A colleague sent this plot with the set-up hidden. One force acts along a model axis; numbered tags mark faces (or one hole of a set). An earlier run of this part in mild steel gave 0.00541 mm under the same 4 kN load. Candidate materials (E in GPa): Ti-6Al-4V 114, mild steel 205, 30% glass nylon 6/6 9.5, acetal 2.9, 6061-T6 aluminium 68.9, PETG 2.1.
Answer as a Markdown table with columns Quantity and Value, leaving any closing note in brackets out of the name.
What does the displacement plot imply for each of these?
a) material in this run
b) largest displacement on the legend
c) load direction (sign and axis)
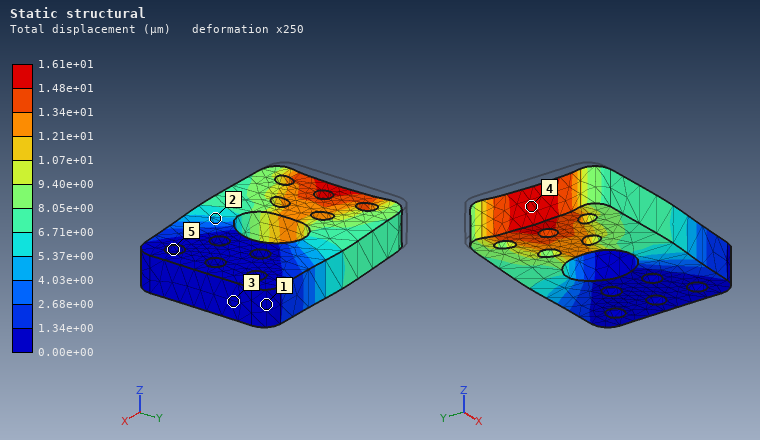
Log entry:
| Quantity | Value |
|---|---|
| material in this run | 6061-T6 aluminium |
| largest displacement on the legend | 1.61e+01 µm |
| load direction | +X |
